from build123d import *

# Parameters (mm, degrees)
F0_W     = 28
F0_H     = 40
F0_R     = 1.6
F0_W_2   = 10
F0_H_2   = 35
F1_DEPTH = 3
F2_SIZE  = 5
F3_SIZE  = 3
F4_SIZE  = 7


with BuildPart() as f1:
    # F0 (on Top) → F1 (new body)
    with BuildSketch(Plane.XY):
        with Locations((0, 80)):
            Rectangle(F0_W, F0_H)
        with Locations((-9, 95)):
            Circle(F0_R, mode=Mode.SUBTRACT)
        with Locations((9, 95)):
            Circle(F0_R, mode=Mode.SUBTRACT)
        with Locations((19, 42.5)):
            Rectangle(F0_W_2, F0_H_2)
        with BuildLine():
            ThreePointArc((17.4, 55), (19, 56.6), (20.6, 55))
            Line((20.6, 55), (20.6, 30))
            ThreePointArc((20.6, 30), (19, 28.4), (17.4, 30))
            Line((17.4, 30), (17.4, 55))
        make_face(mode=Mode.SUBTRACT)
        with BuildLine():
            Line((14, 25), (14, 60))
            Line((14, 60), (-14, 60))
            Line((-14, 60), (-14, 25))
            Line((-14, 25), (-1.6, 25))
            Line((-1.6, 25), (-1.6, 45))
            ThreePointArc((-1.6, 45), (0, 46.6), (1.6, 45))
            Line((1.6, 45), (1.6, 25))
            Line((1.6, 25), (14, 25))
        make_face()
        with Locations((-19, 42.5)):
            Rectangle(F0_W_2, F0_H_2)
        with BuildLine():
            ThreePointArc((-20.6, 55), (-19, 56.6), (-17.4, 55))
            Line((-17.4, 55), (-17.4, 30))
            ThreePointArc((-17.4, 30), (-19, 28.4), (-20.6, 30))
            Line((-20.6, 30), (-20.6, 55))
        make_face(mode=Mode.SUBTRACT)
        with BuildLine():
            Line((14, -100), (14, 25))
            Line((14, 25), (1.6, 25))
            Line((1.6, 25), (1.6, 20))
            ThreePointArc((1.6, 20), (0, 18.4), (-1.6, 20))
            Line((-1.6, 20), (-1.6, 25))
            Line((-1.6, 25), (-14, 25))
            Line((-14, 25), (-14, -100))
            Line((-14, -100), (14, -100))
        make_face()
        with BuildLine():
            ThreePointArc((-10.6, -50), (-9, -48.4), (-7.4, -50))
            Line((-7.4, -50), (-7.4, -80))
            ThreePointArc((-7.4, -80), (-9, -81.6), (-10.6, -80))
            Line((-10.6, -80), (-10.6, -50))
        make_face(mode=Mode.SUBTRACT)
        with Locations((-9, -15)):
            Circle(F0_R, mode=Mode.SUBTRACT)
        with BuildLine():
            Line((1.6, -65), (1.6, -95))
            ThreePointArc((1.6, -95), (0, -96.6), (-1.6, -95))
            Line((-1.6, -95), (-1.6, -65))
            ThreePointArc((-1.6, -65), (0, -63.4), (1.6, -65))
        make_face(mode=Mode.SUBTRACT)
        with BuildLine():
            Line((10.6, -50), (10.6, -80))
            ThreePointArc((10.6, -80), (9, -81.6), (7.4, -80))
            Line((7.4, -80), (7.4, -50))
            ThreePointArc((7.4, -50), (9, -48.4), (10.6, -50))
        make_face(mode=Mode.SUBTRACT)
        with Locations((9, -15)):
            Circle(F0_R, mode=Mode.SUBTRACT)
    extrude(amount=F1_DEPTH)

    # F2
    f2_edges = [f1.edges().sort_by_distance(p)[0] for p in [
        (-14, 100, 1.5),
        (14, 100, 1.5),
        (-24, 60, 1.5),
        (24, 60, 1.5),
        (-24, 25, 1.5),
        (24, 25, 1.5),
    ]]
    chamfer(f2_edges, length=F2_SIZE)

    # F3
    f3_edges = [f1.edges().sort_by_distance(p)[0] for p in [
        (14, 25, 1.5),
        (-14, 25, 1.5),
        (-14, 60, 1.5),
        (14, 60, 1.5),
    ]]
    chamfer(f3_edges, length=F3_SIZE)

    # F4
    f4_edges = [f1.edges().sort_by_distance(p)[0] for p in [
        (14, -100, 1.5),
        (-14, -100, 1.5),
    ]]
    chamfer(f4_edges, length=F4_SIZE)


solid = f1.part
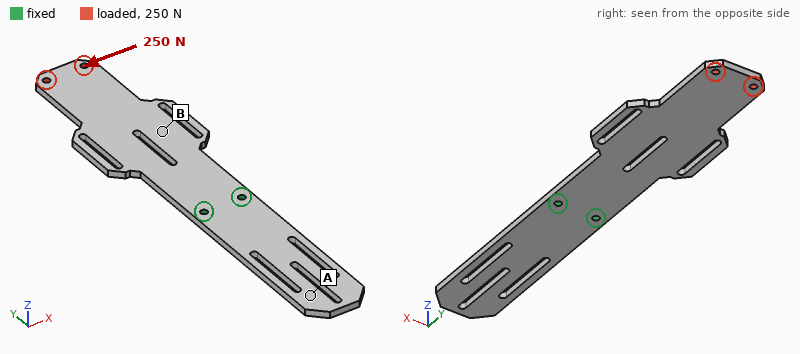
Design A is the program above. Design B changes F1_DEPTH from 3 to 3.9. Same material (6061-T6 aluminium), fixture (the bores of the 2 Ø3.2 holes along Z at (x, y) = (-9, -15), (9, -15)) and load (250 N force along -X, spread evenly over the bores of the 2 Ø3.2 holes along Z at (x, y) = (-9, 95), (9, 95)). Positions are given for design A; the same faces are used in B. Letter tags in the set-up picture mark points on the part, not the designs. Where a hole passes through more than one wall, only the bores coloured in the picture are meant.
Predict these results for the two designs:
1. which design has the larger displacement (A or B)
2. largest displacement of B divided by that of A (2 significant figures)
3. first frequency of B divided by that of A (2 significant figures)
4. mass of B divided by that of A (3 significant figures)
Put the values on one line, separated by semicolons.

A; 0.77; 1.3; 1.30
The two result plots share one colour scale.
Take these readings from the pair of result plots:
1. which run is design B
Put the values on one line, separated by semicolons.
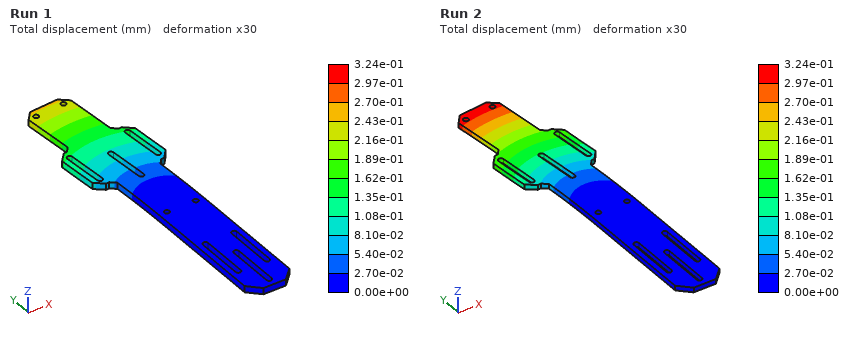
Run 1
